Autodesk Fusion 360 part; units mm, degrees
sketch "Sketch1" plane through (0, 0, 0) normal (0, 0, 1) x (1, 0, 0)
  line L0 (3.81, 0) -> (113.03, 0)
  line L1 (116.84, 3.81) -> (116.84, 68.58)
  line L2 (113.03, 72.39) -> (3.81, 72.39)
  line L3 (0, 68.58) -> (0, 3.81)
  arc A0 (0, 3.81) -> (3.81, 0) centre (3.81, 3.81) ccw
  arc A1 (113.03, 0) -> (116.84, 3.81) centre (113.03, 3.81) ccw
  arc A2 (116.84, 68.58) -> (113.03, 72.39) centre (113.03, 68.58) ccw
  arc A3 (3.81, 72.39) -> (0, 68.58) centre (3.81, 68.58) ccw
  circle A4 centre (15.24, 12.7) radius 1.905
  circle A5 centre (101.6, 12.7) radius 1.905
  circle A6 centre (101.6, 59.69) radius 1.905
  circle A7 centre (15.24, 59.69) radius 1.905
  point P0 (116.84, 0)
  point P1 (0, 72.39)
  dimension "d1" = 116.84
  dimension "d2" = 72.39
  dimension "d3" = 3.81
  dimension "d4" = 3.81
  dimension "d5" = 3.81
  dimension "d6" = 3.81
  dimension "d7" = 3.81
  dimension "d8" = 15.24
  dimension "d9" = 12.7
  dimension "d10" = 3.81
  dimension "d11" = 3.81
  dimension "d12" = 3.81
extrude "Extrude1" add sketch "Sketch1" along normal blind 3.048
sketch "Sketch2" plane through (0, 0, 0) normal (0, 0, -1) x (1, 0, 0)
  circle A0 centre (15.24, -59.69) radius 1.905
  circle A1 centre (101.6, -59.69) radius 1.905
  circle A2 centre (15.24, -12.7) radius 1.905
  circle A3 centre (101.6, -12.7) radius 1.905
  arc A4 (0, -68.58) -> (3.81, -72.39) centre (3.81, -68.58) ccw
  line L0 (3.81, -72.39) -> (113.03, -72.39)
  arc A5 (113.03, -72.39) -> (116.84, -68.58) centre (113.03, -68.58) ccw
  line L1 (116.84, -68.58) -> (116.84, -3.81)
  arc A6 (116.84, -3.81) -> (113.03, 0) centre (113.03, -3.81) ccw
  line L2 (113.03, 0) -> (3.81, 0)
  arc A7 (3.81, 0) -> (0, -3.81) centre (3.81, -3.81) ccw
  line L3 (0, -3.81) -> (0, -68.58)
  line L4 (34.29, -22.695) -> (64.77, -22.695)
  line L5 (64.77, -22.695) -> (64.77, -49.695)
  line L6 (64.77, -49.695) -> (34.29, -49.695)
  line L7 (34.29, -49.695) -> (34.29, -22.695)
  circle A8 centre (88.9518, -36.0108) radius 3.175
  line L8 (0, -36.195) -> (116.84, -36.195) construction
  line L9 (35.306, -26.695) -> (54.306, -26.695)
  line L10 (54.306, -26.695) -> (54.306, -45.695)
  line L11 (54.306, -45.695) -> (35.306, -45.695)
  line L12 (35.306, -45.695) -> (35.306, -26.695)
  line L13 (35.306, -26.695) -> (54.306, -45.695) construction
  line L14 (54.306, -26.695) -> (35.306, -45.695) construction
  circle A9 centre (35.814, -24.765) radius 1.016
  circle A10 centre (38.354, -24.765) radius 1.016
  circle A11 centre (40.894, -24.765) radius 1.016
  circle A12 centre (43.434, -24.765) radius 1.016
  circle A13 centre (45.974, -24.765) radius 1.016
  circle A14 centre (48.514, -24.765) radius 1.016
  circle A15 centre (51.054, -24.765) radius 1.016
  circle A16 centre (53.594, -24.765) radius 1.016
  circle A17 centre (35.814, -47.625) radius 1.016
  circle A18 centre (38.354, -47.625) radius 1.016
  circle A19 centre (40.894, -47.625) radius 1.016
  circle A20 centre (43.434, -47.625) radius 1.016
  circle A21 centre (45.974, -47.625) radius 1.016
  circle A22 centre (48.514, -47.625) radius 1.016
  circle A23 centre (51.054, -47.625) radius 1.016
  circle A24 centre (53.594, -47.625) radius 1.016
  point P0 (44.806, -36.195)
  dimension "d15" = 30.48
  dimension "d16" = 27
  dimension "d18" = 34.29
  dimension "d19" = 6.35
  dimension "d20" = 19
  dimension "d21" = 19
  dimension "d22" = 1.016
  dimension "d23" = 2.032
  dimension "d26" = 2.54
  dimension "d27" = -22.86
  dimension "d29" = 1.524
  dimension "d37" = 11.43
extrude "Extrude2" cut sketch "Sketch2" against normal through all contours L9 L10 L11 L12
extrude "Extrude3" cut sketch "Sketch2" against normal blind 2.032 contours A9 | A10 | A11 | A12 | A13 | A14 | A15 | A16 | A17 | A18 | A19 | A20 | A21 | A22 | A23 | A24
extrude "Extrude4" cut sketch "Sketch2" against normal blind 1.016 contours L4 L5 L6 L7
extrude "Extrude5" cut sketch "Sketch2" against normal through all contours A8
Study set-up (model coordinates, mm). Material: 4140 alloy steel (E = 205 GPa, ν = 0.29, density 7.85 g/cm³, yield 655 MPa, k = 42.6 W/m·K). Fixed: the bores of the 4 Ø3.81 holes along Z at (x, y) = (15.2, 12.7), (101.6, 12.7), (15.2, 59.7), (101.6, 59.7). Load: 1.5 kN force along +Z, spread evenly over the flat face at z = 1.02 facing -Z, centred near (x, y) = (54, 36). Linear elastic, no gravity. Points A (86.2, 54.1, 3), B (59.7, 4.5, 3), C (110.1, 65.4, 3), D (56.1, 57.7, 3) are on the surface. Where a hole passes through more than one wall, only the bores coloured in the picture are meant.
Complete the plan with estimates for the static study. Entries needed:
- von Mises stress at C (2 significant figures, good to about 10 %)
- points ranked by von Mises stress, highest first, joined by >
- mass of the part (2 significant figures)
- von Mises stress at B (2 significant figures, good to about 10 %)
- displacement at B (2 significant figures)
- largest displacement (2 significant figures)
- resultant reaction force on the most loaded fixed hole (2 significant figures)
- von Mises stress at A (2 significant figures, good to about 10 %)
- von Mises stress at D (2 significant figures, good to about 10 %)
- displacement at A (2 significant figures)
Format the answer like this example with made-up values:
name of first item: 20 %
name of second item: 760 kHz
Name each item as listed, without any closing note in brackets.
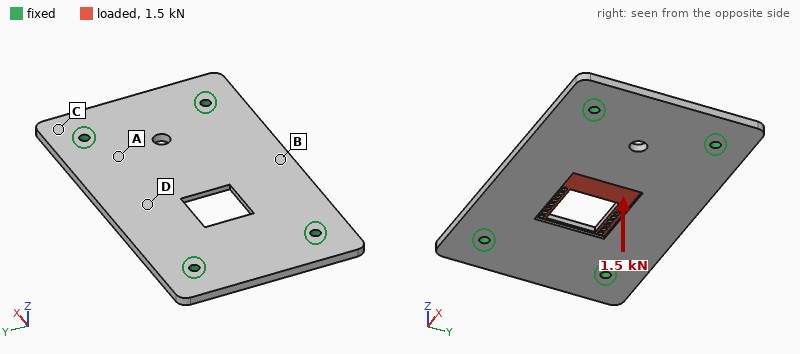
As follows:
von Mises stress at C: 29 MPa
points ranked by von Mises stress, highest first, joined by >: D > B > A > C
mass of the part: 190 g
von Mises stress at B: 100 MPa
displacement at B: 0.13 mm
largest displacement: 0.32 mm
resultant reaction force on the most loaded fixed hole: 480 N
von Mises stress at A: 45 MPa
von Mises stress at D: 130 MPa
displacement at A: 0.064 mm
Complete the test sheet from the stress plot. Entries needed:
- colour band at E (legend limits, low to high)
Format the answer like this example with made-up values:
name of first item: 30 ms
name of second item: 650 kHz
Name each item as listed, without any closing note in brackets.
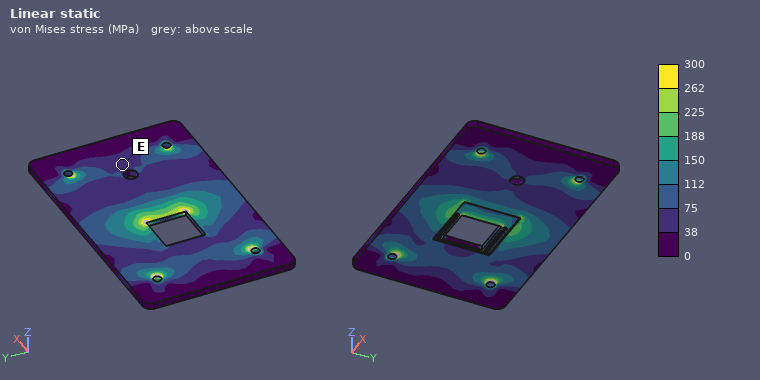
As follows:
colour band at E: 38 to 75 MPa
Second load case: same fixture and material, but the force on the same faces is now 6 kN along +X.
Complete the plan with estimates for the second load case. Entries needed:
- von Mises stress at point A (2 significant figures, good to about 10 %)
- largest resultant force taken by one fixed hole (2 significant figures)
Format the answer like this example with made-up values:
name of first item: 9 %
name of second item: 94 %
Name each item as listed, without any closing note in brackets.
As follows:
von Mises stress at point A: 24 MPa
largest resultant force taken by one fixed hole: 1.7 kN
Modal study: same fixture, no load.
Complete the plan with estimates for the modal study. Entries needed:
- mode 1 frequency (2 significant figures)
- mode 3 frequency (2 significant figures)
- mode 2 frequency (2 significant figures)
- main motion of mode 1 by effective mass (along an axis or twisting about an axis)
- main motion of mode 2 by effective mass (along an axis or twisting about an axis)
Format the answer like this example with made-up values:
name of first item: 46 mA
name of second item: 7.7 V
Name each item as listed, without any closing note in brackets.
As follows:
mode 1 frequency: 2000 Hz
mode 3 frequency: 4200 Hz
mode 2 frequency: 2500 Hz
main motion of mode 1 by effective mass: along Z
main motion of mode 2 by effective mass: twisting about X
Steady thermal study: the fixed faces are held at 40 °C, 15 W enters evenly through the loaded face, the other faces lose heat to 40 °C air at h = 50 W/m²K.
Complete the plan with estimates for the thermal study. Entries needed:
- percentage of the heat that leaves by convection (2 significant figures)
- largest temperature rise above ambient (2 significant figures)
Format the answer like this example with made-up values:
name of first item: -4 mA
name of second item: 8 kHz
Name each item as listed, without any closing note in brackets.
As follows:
percentage of the heat that leaves by convection: 55 %
largest temperature rise above ambient: 46 K
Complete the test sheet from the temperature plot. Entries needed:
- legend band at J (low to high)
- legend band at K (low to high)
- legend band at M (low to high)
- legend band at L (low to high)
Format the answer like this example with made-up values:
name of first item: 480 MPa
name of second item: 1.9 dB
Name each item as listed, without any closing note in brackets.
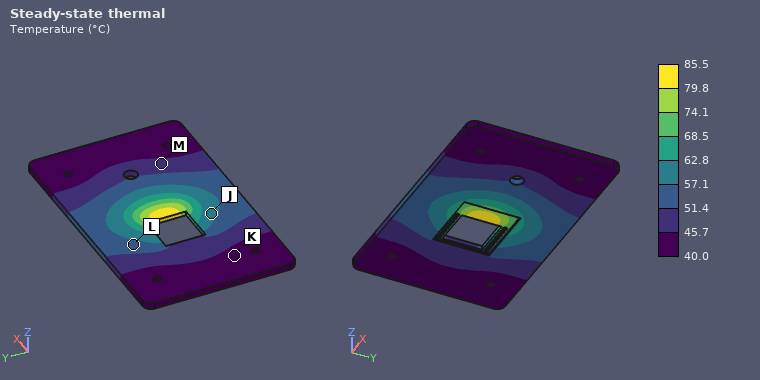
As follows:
legend band at J: 57.1 to 62.8 °C
legend band at K: 40.0 to 45.7 °C
legend band at M: 45.7 to 51.4 °C
legend band at L: 51.4 to 57.1 °C
